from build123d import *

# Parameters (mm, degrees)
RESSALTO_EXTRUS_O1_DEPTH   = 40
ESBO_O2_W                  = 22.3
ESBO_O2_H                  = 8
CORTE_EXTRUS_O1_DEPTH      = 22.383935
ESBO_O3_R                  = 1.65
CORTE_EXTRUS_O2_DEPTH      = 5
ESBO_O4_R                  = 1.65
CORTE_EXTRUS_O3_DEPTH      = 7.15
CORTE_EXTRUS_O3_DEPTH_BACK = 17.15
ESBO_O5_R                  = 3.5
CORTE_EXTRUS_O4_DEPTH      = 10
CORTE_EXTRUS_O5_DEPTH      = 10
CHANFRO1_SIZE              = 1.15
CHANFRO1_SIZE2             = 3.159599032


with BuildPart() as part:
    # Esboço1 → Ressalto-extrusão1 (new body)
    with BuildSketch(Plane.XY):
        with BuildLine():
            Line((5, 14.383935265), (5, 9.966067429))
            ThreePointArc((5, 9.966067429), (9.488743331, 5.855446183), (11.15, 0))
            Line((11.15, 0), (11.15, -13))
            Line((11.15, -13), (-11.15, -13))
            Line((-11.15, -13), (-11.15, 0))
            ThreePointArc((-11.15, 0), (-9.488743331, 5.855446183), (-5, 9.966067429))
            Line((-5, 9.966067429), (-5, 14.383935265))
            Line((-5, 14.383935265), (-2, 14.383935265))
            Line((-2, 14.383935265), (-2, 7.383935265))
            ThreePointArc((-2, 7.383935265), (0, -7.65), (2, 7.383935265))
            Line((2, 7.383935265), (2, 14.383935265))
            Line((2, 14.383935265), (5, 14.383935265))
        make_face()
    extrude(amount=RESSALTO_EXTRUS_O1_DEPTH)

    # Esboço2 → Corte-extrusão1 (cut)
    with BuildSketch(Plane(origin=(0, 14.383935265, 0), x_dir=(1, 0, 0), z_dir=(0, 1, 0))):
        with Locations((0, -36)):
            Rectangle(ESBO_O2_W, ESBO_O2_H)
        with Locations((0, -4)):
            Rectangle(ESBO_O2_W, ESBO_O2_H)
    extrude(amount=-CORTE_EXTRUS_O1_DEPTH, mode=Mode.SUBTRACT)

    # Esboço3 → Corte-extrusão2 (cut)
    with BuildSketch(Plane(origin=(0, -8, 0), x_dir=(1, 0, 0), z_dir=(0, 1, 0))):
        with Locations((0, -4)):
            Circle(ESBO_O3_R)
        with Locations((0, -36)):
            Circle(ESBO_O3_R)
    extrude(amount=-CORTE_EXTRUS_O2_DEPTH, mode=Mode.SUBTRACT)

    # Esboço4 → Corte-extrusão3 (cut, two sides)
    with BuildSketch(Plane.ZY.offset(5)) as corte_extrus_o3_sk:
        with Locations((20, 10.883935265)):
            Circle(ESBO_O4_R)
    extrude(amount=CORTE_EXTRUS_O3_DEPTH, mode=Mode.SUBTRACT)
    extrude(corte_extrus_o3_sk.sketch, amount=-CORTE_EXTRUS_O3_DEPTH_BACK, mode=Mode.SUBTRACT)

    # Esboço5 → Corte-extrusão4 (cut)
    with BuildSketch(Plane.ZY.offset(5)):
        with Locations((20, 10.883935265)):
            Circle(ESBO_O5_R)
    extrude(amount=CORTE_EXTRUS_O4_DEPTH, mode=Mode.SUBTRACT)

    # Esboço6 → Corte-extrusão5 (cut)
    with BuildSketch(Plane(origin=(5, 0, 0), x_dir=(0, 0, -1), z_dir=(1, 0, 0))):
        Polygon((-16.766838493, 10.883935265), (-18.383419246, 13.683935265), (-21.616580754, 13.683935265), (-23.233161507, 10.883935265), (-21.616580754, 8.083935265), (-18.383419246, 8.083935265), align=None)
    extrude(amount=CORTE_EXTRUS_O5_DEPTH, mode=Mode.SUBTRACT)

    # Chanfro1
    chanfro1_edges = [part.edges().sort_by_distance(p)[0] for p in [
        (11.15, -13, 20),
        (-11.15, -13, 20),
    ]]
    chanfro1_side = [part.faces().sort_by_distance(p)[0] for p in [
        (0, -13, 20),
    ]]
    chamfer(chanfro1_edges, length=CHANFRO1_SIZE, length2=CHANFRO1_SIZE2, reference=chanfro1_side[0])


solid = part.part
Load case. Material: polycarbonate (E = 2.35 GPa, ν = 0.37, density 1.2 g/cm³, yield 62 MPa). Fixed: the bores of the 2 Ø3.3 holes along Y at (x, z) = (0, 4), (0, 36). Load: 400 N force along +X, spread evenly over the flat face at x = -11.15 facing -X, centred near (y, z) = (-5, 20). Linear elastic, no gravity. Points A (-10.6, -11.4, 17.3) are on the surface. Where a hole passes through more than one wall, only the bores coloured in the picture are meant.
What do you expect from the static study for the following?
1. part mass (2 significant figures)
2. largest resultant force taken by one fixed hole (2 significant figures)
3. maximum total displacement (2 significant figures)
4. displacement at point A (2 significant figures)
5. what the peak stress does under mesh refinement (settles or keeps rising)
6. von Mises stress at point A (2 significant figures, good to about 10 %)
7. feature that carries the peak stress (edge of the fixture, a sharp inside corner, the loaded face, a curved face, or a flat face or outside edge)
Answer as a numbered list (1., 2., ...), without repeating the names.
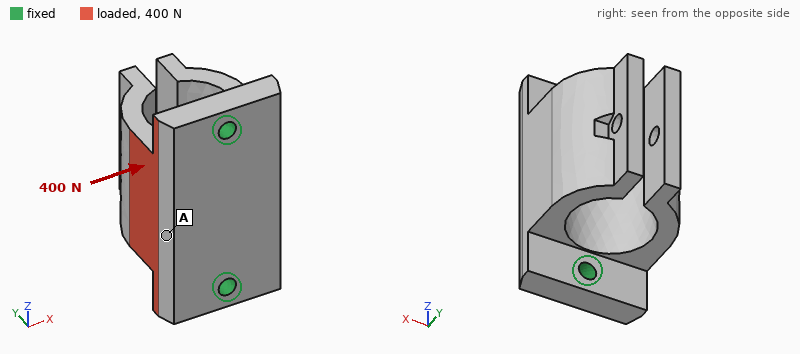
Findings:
1. 11 g
2. 200 N
3. 0.55 mm
4. 0.16 mm
5. keeps rising
6. 4.3 MPa
7. edge of the fixture
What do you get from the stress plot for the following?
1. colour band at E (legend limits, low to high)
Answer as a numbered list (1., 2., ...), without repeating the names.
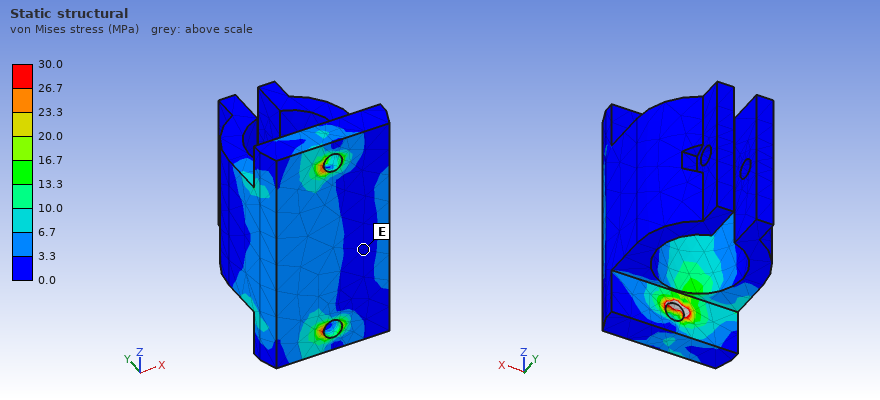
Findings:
1. 0.0 to 3.3 MPa
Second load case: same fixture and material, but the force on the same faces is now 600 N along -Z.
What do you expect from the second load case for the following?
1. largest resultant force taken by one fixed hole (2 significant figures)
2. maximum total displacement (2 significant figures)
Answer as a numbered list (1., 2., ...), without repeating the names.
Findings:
1. 380 N
2. 0.12 mm
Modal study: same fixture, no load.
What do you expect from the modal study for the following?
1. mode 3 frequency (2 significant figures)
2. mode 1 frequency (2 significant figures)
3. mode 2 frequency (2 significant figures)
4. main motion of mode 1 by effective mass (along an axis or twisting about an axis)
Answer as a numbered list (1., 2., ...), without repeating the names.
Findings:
1. 2900 Hz
2. 1400 Hz
3. 1800 Hz
4. along X
